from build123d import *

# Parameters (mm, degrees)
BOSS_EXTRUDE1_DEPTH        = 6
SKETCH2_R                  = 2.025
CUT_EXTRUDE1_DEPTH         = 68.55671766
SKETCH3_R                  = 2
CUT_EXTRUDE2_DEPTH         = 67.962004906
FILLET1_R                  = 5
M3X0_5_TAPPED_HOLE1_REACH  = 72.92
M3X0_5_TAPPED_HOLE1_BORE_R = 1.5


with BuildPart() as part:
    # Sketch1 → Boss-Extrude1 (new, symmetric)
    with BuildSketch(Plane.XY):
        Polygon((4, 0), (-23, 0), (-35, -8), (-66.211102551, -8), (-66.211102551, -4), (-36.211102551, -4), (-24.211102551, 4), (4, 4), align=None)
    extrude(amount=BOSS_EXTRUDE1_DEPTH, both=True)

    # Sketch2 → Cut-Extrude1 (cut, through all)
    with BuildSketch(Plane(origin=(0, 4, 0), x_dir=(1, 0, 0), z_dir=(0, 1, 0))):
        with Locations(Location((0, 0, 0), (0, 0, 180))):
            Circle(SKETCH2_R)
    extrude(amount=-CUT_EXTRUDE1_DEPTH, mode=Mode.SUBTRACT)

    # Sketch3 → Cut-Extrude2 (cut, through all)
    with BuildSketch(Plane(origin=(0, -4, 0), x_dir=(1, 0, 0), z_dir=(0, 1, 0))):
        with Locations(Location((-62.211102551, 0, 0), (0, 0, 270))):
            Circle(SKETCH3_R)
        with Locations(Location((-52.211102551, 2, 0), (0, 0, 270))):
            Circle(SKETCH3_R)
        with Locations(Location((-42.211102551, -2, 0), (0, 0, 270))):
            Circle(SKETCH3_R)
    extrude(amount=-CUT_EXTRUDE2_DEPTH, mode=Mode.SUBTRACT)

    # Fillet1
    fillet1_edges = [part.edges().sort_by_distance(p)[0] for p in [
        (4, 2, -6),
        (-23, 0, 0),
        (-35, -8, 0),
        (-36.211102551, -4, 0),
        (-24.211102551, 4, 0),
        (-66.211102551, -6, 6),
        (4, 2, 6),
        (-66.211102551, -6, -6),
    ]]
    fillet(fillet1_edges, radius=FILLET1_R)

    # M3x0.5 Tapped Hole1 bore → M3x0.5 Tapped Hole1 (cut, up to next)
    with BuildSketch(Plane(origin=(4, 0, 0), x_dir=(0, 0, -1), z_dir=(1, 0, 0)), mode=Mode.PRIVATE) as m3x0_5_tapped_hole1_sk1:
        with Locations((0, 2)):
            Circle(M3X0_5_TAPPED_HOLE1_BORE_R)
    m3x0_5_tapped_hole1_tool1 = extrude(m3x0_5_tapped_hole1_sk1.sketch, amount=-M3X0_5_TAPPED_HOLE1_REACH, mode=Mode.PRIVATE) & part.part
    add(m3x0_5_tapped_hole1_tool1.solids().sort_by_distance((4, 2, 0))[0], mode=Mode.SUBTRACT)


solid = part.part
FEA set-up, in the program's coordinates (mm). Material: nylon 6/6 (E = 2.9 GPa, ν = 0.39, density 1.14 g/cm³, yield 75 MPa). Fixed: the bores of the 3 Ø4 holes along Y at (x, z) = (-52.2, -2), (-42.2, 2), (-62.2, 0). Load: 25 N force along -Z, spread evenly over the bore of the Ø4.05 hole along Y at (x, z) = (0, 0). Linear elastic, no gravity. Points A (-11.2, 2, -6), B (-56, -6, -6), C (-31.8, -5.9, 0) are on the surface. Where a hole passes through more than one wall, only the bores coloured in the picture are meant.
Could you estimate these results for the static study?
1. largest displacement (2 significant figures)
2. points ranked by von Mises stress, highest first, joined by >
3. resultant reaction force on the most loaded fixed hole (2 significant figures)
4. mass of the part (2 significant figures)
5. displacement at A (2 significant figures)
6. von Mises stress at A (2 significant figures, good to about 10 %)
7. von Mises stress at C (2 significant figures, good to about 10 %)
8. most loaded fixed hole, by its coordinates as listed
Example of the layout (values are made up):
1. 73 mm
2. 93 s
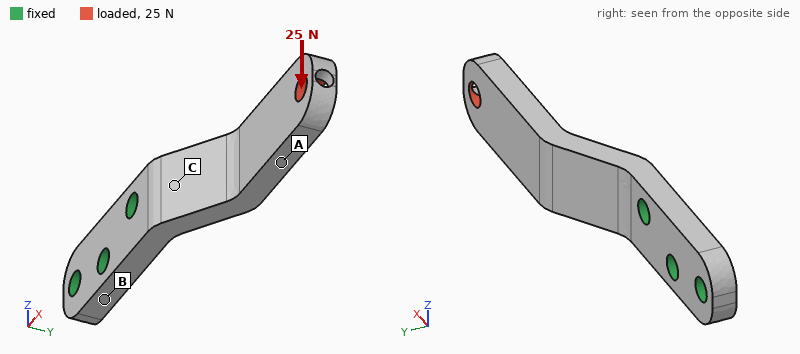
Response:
1. 0.79 mm
2. C > A > B
3. 84 N
4. 3.6 g
5. 0.44 mm
6. 2.9 MPa
7. 8.3 MPa
8. (-42.2, 2)
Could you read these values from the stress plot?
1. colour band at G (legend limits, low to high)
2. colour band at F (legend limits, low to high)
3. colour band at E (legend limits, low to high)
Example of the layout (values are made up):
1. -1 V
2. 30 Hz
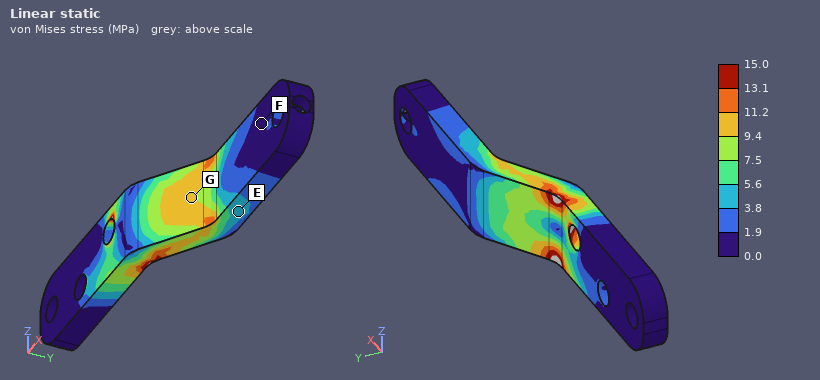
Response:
1. 9.4 to 11.2 MPa
2. 0.0 to 1.9 MPa
3. 3.8 to 5.6 MPa
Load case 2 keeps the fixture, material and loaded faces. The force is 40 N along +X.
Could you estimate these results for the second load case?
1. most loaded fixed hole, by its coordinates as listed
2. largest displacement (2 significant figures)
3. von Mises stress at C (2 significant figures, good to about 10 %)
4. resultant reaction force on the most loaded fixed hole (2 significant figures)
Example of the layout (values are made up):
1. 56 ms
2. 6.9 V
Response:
1. (-42.2, 2)
2. 0.85 mm
3. 6.3 MPa
4. 33 N
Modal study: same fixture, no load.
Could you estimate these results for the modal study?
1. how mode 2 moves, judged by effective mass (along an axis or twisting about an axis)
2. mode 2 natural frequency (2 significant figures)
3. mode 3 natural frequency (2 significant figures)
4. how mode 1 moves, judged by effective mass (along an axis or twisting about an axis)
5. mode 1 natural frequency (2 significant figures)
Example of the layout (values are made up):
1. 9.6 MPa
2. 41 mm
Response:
1. along Z
2. 1100 Hz
3. 2700 Hz
4. along Y
5. 520 Hz
